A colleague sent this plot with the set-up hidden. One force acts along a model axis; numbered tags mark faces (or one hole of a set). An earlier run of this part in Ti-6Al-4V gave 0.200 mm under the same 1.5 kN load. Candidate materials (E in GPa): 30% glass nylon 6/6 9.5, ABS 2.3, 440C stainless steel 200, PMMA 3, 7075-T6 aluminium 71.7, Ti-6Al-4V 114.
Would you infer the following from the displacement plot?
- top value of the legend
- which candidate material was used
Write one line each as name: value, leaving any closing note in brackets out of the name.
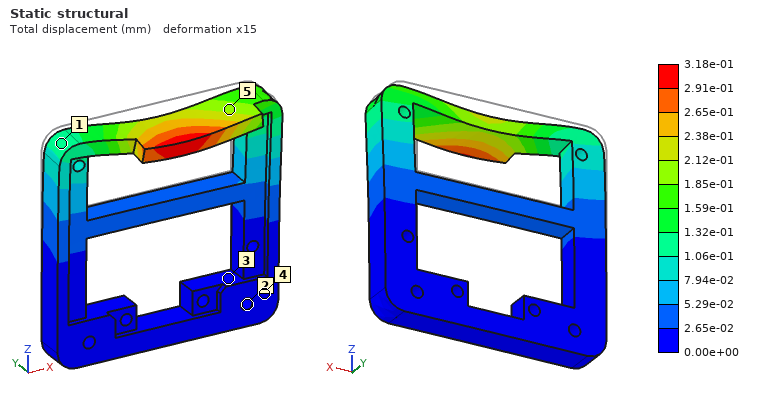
top value of the legend: 3.18e-01 mm
which candidate material was used: 7075-T6 aluminium
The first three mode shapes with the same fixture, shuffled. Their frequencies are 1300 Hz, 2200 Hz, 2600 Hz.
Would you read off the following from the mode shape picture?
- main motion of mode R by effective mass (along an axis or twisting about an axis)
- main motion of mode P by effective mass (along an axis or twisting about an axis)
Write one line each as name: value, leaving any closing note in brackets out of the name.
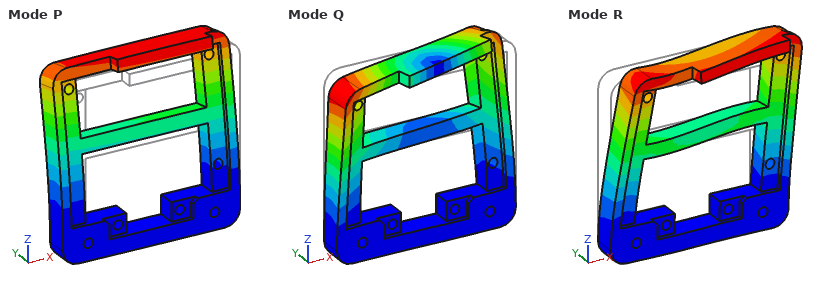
main motion of mode R by effective mass: along X
main motion of mode P by effective mass: along Y
